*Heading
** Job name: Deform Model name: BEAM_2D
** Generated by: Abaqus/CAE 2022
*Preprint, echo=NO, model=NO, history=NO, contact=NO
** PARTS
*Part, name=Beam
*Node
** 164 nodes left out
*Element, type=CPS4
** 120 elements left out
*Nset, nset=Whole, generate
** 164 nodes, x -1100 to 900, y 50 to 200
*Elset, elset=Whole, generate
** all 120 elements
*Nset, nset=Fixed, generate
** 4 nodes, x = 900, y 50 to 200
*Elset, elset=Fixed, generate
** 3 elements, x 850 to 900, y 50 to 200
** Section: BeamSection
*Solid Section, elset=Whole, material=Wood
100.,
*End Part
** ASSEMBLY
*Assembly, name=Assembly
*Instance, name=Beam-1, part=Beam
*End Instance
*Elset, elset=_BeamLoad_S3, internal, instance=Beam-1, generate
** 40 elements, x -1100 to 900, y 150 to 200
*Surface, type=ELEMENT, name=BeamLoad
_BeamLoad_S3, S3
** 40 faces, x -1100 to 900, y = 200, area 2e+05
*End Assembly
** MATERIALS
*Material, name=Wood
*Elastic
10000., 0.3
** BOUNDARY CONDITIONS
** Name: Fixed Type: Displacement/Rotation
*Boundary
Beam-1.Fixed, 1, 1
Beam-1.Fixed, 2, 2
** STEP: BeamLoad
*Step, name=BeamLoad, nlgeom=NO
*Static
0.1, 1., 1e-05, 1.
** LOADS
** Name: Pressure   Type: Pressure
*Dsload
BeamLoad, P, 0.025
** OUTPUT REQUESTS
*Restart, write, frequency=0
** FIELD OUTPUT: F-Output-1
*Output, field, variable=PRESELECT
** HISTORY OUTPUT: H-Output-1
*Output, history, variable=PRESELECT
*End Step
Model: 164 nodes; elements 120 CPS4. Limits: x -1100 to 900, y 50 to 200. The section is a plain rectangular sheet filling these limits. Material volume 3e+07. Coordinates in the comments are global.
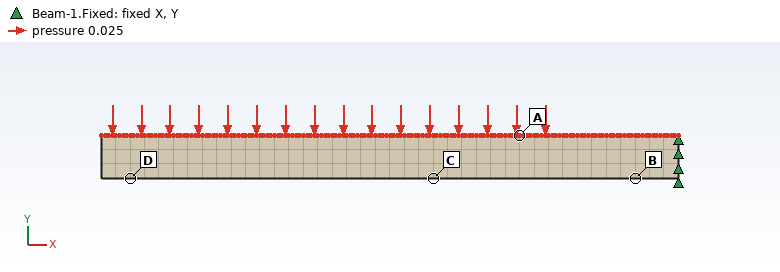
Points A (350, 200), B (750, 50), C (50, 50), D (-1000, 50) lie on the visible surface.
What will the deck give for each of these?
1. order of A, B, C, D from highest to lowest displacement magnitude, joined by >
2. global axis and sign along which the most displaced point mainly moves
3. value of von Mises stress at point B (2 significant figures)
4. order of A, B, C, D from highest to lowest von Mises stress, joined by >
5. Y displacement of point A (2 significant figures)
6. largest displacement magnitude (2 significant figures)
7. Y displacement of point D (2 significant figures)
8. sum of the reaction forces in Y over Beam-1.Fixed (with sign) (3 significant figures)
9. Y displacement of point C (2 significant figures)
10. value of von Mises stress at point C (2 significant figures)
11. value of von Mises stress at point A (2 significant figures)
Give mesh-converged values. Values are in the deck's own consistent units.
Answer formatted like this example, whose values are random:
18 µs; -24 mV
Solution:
D > C > A > B; -Y; 11; B > A > C > D; -2.2; 18; -16; 5000; -4.8; 4.3; 6.9
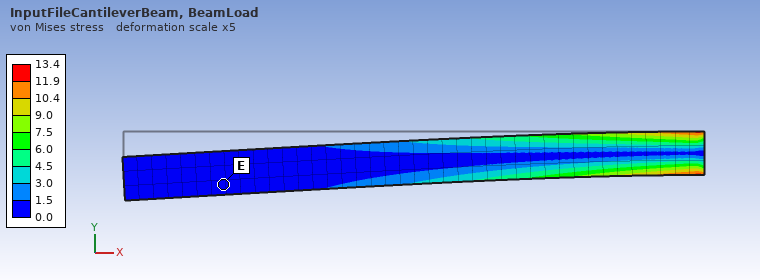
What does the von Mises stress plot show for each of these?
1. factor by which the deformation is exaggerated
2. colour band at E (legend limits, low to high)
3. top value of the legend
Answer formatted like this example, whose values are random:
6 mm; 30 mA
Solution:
5; 0.0 to 1.5; 13.4
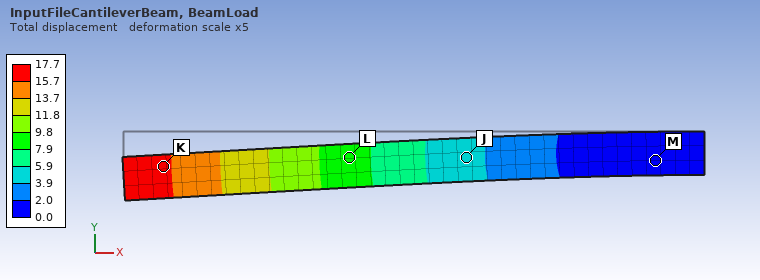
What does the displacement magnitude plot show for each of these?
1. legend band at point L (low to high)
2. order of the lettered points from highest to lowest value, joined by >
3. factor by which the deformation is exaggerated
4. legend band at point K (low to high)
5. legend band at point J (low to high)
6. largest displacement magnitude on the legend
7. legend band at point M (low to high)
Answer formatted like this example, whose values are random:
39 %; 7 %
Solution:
7.9 to 9.8; K > L > J > M; 5; 15.7 to 17.7; 3.9 to 5.9; 17.7; 0.0 to 2.0
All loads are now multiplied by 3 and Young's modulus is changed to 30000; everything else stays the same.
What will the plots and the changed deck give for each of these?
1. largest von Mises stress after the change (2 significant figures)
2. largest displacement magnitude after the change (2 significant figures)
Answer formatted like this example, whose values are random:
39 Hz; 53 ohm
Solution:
40; 18
